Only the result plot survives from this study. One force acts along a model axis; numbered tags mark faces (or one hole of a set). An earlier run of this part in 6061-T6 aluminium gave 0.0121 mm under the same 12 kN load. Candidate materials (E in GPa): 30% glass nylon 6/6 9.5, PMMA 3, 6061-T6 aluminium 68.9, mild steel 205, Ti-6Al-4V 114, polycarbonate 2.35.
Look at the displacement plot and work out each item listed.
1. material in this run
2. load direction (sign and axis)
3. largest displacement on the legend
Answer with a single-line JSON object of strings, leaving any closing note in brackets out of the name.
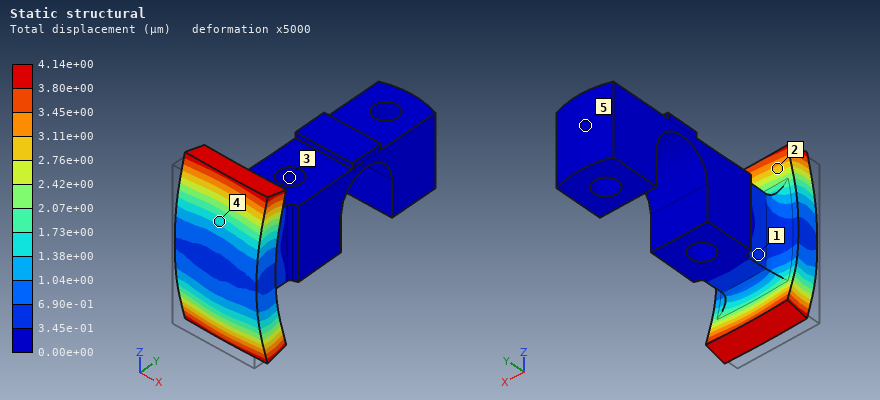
{"material in this run": "mild steel", "load direction": "+Y", "largest displacement on the legend": "4.14e+00 µm"}
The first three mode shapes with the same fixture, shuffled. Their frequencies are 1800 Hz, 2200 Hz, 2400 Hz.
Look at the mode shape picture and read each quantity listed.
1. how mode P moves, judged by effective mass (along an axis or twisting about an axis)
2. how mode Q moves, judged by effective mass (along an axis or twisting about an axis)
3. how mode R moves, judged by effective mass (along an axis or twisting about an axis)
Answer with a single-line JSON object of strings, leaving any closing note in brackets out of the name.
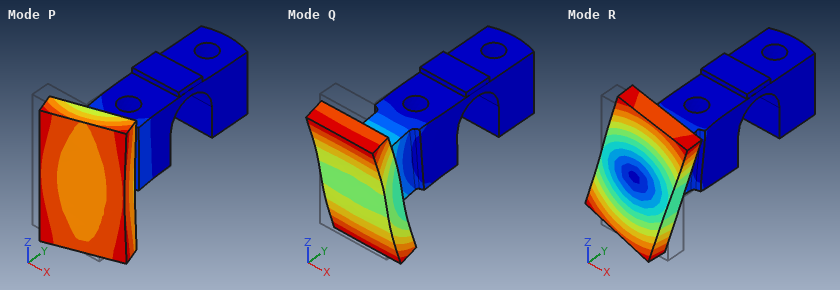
{"how mode P moves, judged by effective mass": "along X", "how mode Q moves, judged by effective mass": "along Z", "how mode R moves, judged by effective mass": "twisting about Y"}
